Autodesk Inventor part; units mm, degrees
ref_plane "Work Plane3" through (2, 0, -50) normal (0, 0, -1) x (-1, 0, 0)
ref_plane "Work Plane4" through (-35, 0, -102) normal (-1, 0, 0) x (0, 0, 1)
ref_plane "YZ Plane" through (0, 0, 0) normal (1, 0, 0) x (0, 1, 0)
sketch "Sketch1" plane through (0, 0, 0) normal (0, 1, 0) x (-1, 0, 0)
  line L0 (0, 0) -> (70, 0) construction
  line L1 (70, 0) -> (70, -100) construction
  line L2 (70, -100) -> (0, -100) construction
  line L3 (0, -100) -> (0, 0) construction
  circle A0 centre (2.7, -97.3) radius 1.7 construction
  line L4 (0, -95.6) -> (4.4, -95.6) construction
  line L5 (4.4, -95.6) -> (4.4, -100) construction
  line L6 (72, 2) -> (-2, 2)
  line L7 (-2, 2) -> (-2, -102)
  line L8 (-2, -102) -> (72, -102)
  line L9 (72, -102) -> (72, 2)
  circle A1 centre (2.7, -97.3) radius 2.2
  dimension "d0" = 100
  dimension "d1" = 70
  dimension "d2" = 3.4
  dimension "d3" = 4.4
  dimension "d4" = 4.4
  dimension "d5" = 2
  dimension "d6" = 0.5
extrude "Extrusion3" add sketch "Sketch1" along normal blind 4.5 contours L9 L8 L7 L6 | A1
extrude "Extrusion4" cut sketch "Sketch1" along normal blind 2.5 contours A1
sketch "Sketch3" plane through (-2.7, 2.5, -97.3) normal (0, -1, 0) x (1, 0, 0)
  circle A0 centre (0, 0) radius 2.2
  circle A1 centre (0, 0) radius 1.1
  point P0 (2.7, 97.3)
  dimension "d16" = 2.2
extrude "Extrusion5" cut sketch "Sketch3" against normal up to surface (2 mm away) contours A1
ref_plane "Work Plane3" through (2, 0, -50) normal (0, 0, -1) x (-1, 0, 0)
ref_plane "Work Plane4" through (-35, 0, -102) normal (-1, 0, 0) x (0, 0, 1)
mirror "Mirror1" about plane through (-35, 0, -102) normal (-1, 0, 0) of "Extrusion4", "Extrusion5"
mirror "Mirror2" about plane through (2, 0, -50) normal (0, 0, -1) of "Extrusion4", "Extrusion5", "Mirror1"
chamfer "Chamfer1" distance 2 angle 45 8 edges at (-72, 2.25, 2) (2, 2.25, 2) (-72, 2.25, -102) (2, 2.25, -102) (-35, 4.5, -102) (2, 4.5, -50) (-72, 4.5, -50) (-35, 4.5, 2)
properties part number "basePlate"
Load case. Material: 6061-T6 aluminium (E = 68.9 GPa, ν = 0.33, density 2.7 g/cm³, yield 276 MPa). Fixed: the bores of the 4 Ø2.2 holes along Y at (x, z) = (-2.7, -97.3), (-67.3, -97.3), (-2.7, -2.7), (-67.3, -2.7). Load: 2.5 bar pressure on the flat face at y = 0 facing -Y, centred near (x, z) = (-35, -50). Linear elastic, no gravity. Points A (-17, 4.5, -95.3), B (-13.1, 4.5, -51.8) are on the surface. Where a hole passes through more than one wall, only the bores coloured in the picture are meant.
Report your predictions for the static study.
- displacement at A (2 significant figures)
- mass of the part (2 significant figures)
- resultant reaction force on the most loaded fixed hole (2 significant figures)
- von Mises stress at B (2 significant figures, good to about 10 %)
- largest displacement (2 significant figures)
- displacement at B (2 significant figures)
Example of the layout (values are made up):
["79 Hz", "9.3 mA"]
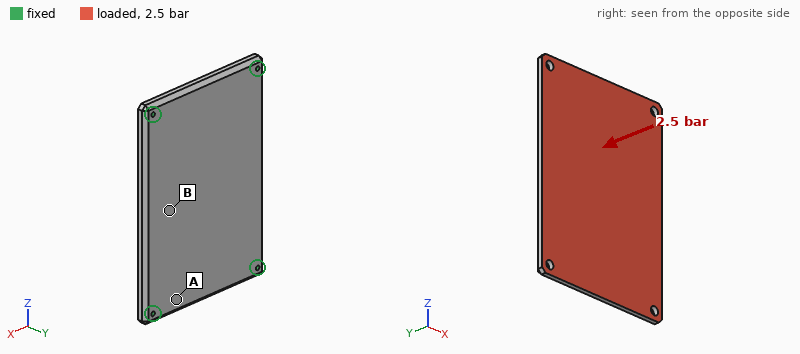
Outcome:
["0.057 mm", "91 g", "1.1 kN", "42 MPa", "0.29 mm", "0.27 mm"]
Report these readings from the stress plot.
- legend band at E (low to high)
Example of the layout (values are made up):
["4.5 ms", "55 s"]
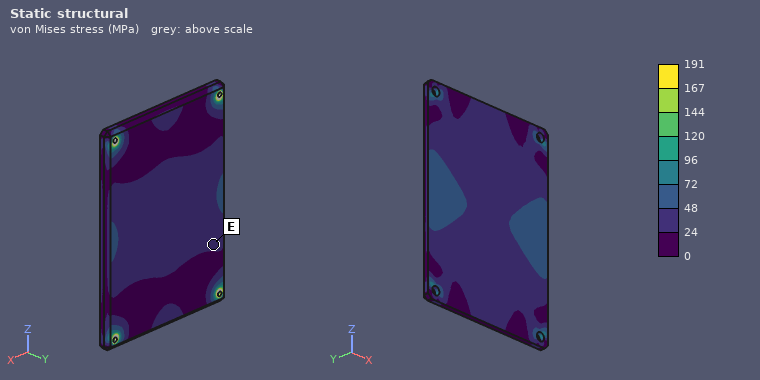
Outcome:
["24 to 48 MPa"]
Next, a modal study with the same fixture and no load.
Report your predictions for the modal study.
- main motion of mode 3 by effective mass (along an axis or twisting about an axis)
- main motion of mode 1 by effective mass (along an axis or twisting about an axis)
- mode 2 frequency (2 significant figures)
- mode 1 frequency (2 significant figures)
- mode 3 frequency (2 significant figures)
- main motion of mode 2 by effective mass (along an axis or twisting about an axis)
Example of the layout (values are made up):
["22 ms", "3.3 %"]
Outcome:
["twisting about X", "along Y", "2800 Hz", "1500 Hz", "3800 Hz", "twisting about Z"]
